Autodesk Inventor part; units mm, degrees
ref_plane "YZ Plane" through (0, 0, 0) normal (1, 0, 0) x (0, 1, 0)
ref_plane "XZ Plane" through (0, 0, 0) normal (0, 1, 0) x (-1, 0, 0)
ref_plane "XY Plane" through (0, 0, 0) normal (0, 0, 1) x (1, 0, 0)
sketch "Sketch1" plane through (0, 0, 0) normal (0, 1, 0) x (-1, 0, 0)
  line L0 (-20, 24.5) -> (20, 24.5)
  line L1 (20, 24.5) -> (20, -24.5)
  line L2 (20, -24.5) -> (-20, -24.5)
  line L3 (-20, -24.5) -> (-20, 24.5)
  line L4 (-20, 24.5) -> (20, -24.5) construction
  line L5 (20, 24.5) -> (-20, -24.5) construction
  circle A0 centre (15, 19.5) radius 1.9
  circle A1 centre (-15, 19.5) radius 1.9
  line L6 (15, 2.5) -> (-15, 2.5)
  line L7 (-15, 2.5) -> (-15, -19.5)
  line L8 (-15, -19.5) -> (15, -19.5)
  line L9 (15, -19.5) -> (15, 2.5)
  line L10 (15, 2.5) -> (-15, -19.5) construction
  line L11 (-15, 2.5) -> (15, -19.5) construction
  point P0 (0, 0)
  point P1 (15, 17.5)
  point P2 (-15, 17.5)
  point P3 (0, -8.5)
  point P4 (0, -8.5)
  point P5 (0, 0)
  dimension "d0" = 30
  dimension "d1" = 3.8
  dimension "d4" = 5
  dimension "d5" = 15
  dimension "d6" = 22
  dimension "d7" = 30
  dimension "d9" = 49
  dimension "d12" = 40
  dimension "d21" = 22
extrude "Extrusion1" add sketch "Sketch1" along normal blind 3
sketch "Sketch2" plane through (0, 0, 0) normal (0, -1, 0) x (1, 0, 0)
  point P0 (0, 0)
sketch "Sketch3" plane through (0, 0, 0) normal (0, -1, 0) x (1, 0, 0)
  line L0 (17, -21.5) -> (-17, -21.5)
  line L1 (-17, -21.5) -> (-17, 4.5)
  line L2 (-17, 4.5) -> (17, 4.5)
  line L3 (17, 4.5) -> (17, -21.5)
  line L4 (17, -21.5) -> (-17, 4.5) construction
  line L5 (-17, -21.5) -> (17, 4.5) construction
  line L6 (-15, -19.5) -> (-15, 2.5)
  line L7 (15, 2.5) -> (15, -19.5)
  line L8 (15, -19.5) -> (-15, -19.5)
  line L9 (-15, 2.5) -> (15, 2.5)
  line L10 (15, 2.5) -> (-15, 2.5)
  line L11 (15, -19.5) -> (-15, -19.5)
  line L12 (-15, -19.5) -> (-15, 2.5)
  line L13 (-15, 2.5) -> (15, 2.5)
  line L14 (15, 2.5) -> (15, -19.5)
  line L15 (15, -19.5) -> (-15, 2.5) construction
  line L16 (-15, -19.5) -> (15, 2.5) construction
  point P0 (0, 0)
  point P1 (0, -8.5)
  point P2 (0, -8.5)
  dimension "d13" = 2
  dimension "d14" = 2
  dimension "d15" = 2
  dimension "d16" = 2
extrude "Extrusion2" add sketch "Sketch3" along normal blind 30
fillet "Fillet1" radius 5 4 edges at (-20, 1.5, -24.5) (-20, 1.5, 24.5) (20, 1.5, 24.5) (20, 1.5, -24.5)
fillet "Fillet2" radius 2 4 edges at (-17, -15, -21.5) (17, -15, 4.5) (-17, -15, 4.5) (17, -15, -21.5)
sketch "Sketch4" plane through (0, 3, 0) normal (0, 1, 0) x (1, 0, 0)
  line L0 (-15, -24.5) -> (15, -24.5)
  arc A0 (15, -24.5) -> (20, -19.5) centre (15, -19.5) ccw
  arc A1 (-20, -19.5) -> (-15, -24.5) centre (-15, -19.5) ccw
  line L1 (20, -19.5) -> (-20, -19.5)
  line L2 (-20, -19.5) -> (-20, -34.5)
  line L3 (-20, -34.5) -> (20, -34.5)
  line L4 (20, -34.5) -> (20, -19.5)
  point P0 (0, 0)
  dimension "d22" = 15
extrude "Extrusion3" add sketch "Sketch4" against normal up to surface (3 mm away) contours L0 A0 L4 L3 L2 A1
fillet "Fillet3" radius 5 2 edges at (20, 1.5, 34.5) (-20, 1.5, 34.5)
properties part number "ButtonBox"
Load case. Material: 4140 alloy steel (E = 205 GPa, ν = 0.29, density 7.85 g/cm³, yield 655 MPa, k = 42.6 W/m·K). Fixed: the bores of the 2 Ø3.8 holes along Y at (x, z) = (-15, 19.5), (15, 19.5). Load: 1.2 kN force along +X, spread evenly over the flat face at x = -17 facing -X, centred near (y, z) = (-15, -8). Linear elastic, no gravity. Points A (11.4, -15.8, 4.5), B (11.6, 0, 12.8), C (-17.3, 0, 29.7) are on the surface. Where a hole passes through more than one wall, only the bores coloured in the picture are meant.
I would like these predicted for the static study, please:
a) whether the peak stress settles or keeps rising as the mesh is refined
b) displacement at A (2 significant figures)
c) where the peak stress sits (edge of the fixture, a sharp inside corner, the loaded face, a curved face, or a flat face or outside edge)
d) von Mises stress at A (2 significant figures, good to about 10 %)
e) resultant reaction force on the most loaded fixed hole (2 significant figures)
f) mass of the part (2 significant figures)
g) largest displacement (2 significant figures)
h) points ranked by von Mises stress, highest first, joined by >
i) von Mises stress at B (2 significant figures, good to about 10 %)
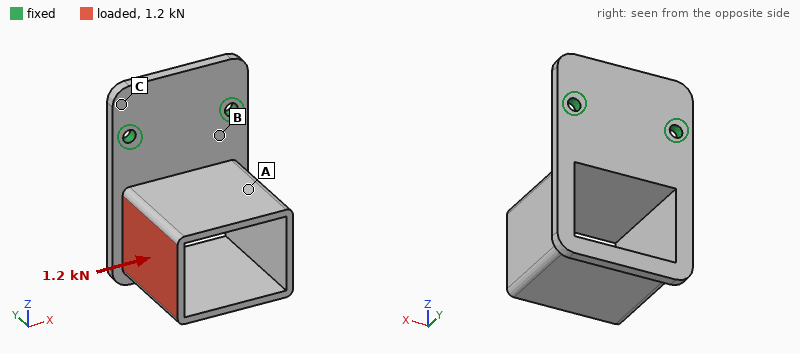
keeps rising
0.076 mm
edge of the fixture
69 MPa
1.4 kN
91 g
0.21 mm
B > A > C
140 MPa
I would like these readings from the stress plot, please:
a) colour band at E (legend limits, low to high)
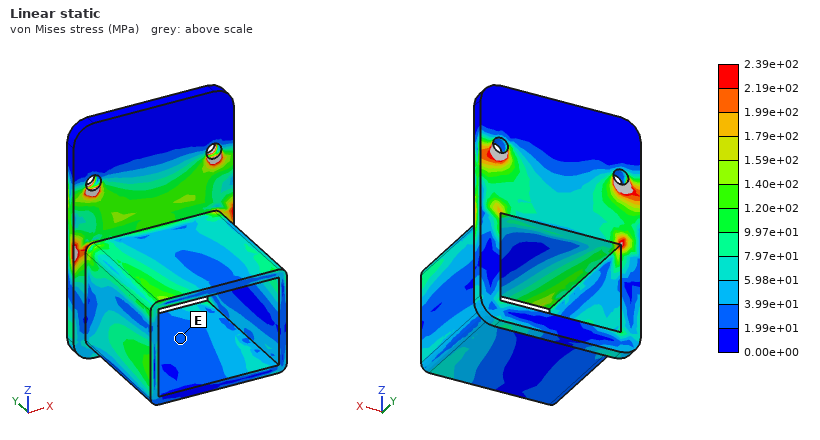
1.99e+01 to 3.99e+01 MPa
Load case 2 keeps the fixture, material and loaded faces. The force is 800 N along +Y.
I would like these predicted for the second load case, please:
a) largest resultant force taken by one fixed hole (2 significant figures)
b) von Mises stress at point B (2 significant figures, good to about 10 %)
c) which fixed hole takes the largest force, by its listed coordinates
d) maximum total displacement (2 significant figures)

850 N
240 MPa
(-15, 19.5)
0.87 mm
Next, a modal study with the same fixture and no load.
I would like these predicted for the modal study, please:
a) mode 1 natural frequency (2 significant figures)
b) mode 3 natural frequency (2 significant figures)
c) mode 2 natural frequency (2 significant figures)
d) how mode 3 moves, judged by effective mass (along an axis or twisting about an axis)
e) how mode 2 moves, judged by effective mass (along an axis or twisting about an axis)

660 Hz
3000 Hz
1900 Hz
along X
along X
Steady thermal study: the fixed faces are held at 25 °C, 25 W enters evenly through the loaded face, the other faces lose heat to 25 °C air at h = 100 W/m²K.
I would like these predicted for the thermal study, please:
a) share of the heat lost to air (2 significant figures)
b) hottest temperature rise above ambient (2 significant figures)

85 %
79 K
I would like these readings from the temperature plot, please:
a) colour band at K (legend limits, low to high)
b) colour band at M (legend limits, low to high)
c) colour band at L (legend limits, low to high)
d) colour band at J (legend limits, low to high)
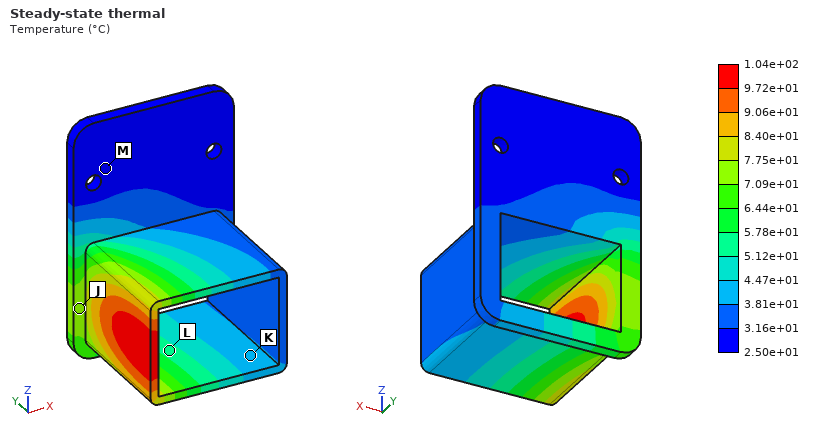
3.81e+01 to 4.47e+01 °C
2.50e+01 to 3.16e+01 °C
5.12e+01 to 5.78e+01 °C
7.09e+01 to 7.75e+01 °C
